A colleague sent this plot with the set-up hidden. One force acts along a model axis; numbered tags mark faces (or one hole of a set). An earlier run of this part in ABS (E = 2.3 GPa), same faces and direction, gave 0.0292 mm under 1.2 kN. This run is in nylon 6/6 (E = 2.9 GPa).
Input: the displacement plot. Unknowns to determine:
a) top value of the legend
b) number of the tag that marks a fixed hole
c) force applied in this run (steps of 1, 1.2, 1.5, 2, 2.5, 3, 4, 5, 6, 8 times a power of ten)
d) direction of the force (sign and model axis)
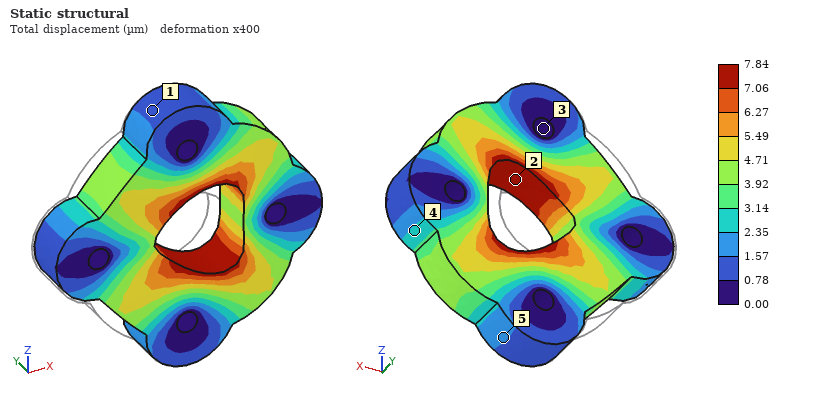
7.84 µm
3
400 N
+X
